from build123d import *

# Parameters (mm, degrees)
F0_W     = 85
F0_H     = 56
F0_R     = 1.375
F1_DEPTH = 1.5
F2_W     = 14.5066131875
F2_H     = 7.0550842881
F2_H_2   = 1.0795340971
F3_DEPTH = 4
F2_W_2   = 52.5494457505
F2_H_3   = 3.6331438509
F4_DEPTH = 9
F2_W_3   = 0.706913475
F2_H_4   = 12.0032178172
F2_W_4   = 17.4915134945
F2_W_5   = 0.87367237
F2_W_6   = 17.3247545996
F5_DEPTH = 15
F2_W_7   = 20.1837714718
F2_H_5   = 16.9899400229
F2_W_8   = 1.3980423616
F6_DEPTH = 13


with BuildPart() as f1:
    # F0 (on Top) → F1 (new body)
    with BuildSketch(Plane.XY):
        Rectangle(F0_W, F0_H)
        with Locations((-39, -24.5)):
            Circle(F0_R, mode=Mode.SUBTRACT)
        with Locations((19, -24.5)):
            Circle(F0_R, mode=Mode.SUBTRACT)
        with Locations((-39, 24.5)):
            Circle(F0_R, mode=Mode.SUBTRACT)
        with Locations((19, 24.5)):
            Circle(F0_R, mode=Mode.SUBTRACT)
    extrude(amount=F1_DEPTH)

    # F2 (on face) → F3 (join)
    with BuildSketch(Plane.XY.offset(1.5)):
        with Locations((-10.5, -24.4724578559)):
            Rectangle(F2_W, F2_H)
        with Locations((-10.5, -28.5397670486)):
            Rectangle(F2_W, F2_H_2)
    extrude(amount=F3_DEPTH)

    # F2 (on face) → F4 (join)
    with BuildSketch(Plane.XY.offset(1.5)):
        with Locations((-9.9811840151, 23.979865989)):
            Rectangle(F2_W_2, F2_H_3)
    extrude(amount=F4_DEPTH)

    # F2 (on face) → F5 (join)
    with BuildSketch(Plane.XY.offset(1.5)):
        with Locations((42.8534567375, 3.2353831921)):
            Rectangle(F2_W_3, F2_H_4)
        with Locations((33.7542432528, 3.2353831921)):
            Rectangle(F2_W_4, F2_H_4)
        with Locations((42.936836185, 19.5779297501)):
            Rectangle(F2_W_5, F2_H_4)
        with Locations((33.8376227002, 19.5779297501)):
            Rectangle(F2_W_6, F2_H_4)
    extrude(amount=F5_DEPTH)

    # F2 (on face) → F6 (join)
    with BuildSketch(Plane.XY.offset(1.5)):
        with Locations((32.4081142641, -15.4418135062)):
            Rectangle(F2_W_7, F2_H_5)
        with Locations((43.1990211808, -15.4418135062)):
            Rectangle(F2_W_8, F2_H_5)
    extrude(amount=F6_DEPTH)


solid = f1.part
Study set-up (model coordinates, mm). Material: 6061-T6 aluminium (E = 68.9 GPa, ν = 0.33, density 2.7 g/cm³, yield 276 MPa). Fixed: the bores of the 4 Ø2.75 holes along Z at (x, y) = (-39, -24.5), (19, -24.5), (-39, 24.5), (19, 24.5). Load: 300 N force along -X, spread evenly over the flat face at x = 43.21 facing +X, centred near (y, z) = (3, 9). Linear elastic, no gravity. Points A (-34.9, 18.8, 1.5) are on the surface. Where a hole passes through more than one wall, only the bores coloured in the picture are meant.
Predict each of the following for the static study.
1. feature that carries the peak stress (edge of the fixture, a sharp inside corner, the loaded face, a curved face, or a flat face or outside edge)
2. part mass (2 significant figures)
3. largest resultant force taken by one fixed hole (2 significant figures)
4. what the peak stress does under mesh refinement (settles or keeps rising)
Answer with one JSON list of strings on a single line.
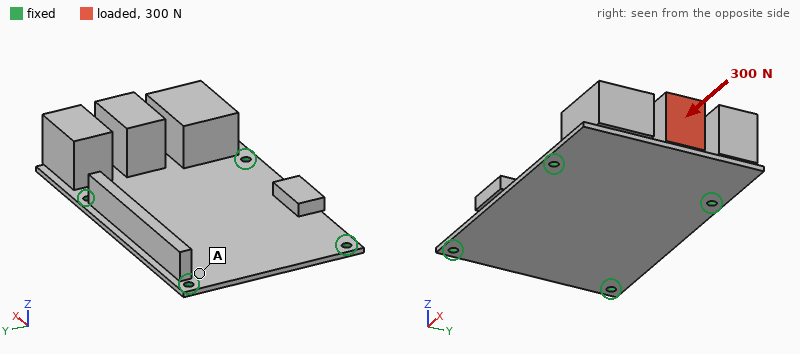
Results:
["edge of the fixture", "56 g", "110 N", "keeps rising"]
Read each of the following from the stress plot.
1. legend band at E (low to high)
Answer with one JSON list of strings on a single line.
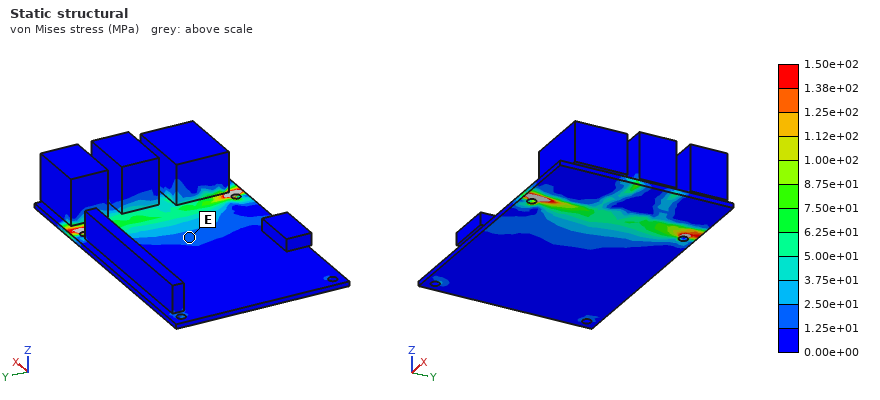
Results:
["1.25e+01 to 2.50e+01 MPa"]
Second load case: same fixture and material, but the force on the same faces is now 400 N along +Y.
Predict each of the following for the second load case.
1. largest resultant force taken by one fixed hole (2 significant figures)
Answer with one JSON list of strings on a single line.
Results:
["290 N"]
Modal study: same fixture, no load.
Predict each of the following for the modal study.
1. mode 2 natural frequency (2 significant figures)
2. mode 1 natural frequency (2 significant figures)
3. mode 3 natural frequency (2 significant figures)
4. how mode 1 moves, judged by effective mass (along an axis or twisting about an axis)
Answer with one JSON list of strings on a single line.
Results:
["1700 Hz", "590 Hz", "2200 Hz", "along Z"]
